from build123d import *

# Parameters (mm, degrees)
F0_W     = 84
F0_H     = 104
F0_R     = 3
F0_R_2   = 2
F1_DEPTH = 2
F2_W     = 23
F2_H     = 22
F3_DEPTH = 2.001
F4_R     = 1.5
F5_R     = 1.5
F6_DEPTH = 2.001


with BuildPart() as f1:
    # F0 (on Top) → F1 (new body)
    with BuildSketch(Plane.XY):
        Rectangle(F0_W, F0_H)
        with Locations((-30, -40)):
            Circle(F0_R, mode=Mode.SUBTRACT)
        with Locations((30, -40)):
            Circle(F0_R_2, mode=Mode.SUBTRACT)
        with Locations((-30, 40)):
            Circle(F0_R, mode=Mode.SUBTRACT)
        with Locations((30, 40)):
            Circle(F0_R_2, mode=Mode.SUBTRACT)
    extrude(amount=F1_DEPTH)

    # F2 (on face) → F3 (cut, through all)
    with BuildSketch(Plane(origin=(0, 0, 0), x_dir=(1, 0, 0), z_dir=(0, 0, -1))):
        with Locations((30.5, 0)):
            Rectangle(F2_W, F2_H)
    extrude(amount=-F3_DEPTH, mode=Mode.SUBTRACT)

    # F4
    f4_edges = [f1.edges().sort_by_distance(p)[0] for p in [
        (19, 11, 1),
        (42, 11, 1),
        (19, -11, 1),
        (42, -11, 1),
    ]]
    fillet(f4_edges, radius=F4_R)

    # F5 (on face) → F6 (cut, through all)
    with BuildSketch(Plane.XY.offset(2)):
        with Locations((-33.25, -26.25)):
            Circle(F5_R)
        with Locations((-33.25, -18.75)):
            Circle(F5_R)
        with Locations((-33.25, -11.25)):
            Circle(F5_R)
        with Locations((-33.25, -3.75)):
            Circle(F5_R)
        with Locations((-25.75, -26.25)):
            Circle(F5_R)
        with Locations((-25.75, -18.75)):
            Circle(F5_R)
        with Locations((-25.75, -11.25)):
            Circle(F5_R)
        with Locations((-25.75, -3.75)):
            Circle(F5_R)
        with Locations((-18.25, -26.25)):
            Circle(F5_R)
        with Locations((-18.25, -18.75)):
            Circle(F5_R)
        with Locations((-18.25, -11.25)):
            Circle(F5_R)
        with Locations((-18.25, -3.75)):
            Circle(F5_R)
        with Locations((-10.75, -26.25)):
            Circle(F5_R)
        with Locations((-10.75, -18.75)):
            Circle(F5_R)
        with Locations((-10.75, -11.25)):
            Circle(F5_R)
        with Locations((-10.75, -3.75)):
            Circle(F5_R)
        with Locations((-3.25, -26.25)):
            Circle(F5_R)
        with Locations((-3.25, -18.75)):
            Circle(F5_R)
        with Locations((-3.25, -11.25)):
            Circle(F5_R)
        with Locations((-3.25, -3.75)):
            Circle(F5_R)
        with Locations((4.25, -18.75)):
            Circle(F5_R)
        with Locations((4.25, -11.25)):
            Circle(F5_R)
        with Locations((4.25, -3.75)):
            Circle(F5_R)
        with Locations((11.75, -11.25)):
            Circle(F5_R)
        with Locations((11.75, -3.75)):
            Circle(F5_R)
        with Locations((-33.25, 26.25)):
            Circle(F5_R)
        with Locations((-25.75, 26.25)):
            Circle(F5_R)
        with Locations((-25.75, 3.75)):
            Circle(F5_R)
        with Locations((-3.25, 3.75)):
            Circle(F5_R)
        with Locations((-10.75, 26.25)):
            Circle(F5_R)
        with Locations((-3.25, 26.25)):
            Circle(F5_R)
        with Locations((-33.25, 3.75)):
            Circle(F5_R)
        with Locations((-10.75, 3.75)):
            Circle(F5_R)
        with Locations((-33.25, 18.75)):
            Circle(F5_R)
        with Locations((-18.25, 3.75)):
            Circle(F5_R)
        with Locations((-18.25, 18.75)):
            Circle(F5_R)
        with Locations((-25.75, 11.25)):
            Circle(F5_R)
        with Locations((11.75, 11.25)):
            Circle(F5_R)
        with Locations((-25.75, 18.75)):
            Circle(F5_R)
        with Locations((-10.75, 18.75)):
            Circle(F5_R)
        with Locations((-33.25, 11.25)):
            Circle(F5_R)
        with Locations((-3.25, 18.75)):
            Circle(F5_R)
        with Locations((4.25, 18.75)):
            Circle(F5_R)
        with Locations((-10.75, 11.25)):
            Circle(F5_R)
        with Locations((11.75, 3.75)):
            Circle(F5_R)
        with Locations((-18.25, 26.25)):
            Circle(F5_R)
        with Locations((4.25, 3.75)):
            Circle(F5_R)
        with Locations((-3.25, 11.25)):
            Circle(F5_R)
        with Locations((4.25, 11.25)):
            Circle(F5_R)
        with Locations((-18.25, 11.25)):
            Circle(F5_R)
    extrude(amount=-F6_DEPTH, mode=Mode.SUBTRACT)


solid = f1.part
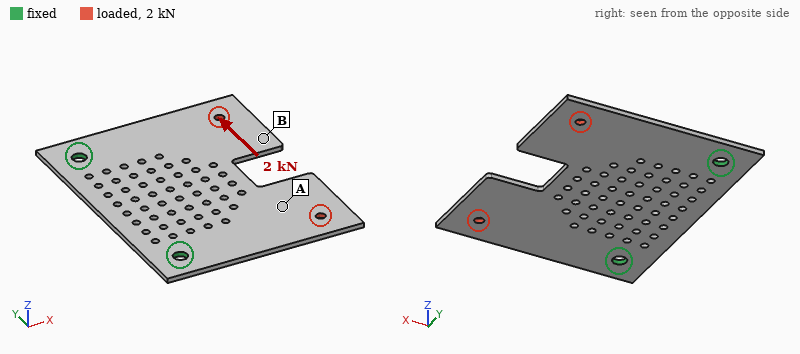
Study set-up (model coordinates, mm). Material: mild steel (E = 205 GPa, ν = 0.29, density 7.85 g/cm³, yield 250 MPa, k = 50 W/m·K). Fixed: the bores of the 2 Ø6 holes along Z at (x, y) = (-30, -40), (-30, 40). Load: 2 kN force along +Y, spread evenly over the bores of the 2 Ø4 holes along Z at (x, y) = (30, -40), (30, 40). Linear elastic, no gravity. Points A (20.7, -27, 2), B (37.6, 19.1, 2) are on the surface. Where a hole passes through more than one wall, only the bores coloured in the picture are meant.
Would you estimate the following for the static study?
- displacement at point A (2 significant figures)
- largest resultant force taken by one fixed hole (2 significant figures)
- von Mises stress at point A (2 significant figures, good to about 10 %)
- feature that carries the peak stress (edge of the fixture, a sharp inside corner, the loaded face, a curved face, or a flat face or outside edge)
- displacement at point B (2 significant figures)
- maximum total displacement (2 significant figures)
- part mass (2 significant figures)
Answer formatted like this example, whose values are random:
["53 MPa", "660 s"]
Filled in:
["16 µm", "1.7 kN", "28 MPa", "a curved face", "22 µm", "26 µm", "120 g"]
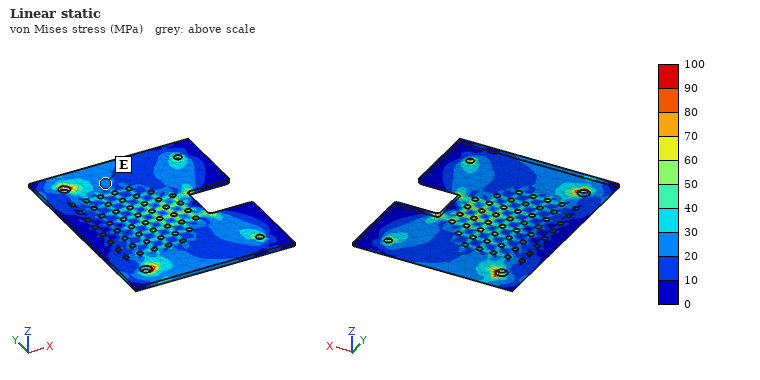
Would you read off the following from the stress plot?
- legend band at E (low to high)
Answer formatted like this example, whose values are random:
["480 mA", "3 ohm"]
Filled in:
["20 to 30 MPa"]
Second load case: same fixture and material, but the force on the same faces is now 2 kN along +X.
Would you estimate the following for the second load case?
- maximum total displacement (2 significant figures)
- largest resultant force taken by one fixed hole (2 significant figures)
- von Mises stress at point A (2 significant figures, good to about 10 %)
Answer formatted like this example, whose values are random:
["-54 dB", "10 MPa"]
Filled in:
["7.4 µm", "1.0 kN", "9.4 MPa"]
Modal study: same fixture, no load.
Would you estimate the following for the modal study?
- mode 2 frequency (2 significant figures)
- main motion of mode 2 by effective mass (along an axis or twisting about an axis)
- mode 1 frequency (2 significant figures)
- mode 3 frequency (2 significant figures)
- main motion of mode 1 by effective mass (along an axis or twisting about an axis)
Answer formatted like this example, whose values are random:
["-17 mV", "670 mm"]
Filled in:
["520 Hz", "twisting about X", "300 Hz", "1100 Hz", "along Z"]
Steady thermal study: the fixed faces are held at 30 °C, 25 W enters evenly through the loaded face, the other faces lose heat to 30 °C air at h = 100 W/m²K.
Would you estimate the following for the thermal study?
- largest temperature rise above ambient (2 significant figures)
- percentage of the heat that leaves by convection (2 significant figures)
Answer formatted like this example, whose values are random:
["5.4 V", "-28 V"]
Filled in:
["75 K", "95 %"]
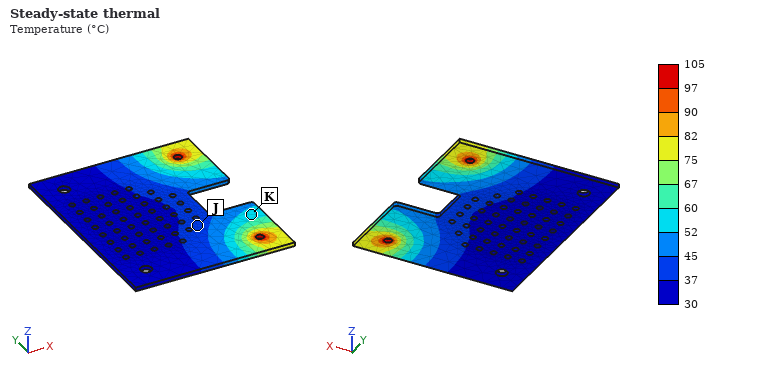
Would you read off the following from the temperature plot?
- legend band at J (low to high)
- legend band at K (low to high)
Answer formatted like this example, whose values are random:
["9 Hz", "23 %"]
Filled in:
["37 to 45 °C", "52 to 60 °C"]
